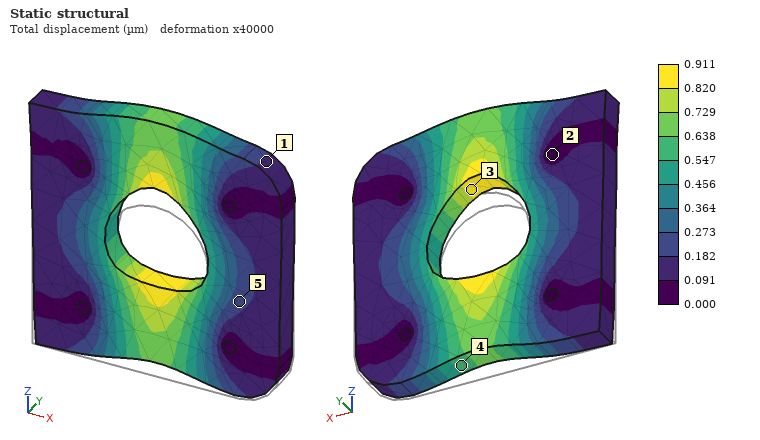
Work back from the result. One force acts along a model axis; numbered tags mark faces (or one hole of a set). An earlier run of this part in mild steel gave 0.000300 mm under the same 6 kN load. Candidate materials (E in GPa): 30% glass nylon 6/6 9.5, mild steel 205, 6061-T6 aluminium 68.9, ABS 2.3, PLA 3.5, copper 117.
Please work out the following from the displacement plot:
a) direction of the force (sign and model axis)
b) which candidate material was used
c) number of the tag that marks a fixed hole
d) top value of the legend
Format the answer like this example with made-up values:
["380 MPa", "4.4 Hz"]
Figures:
["+Z", "6061-T6 aluminium", "2", "0.911 µm"]
